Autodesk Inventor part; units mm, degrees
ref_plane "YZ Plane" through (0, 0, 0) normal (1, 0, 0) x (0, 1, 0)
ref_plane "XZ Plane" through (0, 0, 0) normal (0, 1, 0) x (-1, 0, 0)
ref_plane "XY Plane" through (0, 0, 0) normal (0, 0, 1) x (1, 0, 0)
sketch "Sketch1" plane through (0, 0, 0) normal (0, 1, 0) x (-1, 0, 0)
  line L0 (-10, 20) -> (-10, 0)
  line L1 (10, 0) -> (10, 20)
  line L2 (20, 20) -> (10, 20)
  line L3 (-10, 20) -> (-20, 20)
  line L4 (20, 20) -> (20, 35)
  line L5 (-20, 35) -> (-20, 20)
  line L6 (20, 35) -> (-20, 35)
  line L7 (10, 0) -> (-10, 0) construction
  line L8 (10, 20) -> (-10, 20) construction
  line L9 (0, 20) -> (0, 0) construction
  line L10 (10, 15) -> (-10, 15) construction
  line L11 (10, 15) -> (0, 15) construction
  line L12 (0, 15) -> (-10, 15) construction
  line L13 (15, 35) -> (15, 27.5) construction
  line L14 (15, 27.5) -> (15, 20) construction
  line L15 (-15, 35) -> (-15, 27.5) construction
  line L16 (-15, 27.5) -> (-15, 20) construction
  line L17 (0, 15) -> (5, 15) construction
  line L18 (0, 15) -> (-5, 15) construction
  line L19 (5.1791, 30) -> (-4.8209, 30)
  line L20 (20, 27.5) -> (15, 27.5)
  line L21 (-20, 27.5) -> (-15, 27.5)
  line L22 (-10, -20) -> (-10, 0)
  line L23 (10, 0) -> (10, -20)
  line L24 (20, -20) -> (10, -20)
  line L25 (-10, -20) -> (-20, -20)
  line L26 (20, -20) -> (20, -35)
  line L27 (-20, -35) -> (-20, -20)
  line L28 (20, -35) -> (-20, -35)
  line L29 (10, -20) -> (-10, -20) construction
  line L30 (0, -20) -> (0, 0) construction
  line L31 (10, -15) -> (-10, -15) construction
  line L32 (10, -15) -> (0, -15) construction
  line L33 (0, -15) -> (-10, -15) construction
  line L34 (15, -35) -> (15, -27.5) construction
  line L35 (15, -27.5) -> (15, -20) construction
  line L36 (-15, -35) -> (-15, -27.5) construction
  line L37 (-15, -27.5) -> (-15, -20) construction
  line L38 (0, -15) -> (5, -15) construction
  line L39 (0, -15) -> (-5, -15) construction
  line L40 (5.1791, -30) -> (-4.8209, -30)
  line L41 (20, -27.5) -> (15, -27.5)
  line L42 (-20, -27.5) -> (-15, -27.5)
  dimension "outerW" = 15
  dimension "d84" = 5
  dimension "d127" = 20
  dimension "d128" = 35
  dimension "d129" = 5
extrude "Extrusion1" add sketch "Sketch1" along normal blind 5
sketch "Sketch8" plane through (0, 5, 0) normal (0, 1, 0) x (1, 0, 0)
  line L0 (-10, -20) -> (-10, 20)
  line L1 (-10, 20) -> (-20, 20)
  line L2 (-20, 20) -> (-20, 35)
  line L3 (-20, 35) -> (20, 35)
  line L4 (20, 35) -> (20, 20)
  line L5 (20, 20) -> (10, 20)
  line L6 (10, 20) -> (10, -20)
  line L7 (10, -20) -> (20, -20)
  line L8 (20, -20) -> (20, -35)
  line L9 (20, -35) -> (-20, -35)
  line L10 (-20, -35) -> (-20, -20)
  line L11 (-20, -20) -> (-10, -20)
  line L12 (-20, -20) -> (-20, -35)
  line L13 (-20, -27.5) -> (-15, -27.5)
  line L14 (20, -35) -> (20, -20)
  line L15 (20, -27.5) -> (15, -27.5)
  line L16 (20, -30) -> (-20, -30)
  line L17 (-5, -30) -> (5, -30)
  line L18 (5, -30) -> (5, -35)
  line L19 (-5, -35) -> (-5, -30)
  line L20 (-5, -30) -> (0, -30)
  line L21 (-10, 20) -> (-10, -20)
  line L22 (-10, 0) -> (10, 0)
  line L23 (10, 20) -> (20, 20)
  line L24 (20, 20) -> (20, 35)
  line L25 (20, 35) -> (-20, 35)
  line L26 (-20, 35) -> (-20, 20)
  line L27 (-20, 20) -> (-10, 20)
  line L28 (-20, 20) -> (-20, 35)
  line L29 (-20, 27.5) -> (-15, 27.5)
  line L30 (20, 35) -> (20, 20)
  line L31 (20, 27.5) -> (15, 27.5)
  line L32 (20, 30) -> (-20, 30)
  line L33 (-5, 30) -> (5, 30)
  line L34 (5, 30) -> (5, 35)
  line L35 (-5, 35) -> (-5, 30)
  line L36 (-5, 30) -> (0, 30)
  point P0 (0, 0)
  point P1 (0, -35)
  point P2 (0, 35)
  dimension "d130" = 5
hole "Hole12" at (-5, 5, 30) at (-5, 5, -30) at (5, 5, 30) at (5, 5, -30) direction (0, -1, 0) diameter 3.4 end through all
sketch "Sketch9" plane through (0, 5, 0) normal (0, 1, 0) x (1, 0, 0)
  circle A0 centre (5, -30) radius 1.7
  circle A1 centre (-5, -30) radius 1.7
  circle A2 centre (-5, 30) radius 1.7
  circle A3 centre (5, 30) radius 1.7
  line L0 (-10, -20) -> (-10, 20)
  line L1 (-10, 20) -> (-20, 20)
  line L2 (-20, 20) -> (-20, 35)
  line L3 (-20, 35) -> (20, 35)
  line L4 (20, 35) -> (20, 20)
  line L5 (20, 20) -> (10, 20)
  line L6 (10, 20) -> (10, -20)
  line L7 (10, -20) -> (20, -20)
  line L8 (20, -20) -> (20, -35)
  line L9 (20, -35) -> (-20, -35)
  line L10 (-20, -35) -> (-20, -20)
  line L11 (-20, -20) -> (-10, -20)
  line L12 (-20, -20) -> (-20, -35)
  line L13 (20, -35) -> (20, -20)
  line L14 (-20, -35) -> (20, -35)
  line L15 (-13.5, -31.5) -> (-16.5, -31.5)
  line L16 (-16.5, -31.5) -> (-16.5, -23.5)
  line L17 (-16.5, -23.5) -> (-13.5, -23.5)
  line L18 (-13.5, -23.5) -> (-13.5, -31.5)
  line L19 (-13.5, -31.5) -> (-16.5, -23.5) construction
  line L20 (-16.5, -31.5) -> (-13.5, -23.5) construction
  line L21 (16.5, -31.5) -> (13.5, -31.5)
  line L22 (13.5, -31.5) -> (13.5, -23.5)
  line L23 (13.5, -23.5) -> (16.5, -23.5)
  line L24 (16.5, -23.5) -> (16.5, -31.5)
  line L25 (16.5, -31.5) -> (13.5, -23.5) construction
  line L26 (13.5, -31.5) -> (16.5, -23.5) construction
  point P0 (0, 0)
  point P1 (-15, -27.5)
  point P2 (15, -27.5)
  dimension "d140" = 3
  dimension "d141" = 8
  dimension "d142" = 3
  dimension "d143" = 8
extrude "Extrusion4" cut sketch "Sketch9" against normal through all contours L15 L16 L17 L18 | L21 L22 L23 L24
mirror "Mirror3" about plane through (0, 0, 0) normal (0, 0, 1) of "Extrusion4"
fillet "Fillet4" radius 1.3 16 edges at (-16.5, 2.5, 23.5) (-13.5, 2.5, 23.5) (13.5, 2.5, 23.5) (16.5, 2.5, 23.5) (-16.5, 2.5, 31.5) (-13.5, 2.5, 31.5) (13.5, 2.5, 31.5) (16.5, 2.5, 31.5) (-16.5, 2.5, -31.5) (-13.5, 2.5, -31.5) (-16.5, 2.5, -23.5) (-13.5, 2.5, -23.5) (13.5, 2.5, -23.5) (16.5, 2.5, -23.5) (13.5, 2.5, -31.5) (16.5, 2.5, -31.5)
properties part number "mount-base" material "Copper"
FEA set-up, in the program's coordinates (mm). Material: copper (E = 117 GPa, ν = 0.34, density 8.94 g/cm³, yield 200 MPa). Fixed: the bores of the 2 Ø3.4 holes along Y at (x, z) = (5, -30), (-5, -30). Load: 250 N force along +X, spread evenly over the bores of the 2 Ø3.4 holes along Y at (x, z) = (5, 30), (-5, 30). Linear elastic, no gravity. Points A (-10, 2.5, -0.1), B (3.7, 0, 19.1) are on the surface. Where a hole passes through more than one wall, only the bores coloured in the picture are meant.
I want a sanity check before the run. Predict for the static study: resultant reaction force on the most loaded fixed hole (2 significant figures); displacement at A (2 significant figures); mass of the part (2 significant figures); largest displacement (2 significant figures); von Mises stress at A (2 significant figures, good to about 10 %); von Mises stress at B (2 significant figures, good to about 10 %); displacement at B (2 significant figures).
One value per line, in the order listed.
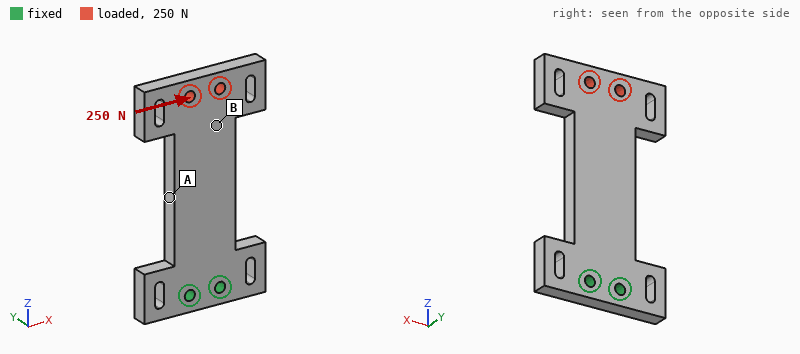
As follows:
1.2 kN
19 µm
84 g
60 µm
23 MPa
6.7 MPa
37 µm
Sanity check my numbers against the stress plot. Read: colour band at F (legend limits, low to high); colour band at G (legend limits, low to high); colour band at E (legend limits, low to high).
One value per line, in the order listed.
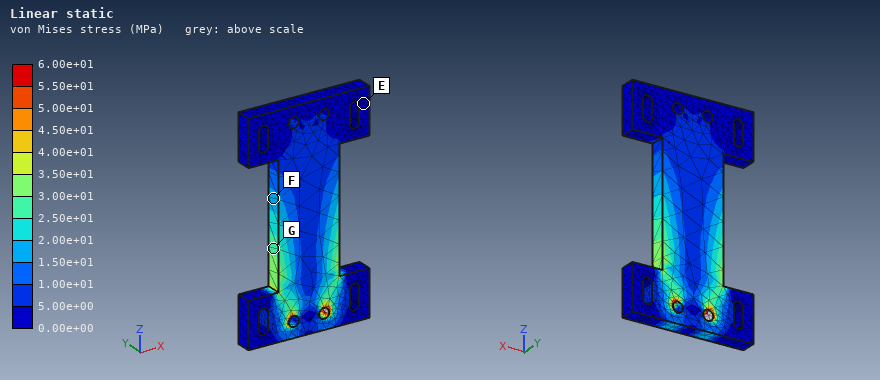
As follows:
1.50e+01 to 2.00e+01 MPa
2.50e+01 to 3.00e+01 MPa
0.00e+00 to 5.00e+00 MPa
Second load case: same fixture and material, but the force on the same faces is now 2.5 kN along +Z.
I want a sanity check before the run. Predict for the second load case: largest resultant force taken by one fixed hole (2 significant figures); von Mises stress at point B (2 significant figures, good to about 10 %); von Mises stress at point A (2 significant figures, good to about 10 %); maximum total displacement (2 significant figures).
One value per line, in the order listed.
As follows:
1.3 kN
25 MPa
25 MPa
14 µm
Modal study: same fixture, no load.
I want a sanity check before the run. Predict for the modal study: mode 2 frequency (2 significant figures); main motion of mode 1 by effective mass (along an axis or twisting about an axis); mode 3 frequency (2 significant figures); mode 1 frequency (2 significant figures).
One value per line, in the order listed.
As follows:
2100 Hz
along Y
2100 Hz
590 Hz
